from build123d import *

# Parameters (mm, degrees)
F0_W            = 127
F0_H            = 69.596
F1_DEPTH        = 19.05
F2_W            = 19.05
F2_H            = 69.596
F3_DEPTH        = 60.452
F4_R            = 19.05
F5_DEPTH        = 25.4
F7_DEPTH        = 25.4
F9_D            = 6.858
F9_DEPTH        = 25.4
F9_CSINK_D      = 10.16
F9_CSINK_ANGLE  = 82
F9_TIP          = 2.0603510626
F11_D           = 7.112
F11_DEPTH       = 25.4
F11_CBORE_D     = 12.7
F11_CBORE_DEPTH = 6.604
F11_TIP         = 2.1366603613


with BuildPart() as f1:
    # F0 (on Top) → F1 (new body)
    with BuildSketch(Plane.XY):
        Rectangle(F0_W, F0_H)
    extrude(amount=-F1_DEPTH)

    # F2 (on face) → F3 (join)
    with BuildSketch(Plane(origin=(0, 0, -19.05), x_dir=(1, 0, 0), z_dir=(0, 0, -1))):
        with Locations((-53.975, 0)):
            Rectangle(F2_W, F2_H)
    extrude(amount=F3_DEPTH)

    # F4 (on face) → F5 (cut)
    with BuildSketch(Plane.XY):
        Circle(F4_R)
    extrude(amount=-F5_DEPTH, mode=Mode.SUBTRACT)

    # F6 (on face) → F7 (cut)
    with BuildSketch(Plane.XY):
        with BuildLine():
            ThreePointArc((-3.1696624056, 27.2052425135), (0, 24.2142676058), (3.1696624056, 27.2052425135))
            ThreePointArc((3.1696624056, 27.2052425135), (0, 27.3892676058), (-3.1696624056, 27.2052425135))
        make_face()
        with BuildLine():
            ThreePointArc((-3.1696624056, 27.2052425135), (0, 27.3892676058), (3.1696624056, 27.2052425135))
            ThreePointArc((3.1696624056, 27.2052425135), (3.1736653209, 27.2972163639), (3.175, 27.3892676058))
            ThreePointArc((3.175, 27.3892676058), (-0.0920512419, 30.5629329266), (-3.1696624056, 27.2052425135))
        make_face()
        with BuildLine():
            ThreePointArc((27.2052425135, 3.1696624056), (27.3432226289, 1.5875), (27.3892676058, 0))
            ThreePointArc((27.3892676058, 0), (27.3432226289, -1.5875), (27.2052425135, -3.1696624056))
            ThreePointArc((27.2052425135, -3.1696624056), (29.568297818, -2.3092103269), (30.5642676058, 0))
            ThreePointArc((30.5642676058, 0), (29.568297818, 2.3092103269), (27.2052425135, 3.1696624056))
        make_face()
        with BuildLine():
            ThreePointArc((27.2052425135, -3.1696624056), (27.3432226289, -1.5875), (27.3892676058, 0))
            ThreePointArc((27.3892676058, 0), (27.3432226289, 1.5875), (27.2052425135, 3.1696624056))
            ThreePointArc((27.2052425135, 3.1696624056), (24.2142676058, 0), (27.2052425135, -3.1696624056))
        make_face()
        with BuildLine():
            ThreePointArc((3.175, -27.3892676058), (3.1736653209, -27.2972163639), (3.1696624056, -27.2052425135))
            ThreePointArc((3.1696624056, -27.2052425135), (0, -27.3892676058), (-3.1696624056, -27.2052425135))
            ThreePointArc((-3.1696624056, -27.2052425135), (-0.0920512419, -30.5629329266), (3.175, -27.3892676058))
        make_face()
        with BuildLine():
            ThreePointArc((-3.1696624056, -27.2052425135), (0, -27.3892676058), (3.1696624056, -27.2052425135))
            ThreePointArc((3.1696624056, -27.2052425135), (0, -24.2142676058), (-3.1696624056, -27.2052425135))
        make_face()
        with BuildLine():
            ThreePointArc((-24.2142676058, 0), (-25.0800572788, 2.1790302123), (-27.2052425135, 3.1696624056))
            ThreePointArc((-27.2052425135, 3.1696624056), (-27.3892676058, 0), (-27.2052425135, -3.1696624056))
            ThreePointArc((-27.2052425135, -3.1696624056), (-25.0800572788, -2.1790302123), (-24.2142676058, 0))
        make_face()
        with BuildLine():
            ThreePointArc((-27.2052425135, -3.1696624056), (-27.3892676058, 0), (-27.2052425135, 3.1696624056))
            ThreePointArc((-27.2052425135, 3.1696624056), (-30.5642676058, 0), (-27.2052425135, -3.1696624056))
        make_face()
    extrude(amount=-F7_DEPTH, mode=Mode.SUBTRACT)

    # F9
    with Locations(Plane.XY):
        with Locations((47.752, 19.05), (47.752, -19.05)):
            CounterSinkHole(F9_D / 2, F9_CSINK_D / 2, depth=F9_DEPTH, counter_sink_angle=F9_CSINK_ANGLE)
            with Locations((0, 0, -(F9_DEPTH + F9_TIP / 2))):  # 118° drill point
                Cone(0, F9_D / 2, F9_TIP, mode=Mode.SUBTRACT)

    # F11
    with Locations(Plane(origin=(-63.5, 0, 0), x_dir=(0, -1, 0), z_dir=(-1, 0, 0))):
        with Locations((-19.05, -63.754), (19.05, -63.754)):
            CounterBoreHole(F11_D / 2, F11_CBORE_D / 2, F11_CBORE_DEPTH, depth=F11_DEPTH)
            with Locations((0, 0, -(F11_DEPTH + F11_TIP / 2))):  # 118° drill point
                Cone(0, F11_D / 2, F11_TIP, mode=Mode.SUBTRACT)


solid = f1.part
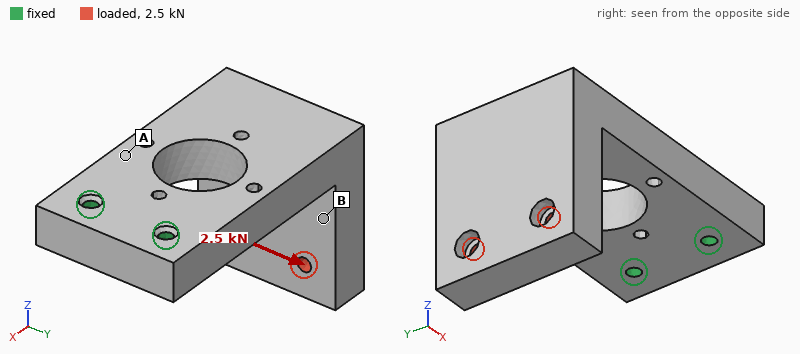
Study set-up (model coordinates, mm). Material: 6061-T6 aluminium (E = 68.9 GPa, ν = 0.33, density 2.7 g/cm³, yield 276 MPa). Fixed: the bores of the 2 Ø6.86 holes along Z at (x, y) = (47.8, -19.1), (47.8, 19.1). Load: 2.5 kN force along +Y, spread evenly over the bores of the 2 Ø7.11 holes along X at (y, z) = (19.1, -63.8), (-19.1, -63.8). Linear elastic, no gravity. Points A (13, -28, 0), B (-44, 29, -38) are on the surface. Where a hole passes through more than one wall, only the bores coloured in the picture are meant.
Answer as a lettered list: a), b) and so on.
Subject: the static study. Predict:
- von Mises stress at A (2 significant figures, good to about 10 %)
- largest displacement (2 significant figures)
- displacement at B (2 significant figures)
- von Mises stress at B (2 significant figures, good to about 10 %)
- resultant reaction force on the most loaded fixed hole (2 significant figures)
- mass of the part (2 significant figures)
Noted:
a) 38 MPa
b) 0.44 mm
c) 0.24 mm
d) 10 MPa
e) 6.4 kN
f) 590 g
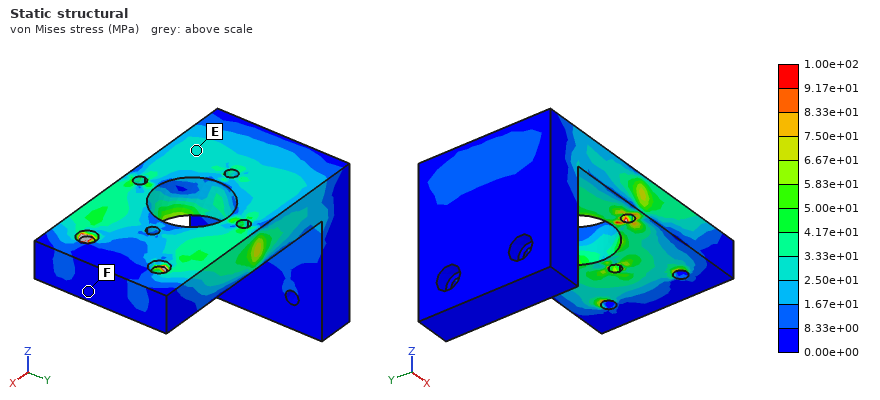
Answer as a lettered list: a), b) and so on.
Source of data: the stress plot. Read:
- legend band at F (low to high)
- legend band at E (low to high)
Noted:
a) 0.00e+00 to 8.33e+00 MPa
b) 2.50e+01 to 3.33e+01 MPa
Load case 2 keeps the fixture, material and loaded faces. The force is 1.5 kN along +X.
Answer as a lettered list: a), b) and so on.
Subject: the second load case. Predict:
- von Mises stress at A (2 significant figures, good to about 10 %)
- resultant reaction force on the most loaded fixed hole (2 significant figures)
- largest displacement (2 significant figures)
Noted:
a) 31 MPa
b) 750 N
c) 0.48 mm
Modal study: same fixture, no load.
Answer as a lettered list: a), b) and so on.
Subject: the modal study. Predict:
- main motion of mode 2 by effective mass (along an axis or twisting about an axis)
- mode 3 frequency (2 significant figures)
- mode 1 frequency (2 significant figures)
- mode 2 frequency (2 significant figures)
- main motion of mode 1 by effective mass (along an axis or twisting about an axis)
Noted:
a) along Y
b) 2100 Hz
c) 530 Hz
d) 1000 Hz
e) along Z
